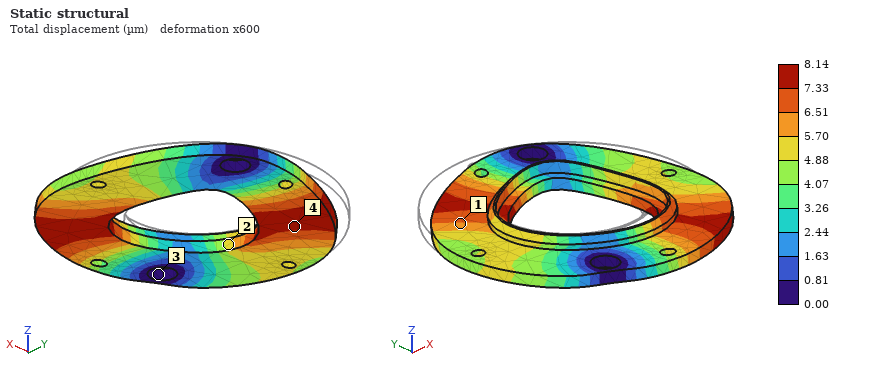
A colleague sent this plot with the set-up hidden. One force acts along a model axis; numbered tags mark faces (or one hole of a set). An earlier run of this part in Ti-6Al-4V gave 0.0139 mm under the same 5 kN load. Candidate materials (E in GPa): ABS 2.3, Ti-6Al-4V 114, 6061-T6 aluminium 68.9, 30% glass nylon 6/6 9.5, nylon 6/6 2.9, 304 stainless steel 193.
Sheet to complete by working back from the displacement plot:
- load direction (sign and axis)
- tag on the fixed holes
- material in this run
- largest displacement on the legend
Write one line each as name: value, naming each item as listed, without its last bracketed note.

load direction: -Y
tag on the fixed holes: 3
material in this run: 304 stainless steel
largest displacement on the legend: 8.14 µm
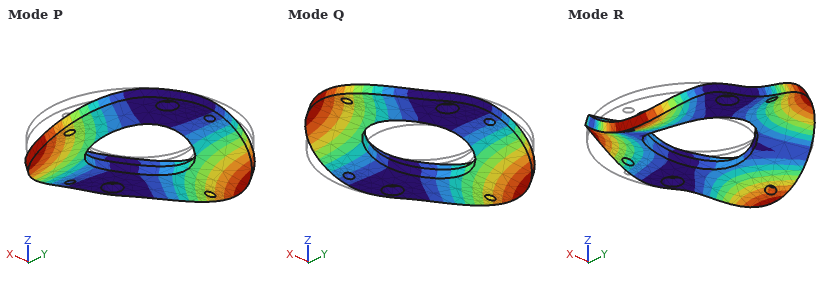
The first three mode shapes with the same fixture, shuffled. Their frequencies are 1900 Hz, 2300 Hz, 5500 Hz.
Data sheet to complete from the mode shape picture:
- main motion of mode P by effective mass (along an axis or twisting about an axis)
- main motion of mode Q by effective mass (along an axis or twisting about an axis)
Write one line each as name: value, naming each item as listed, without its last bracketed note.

main motion of mode P by effective mass: along Z
main motion of mode Q by effective mass: twisting about Y
